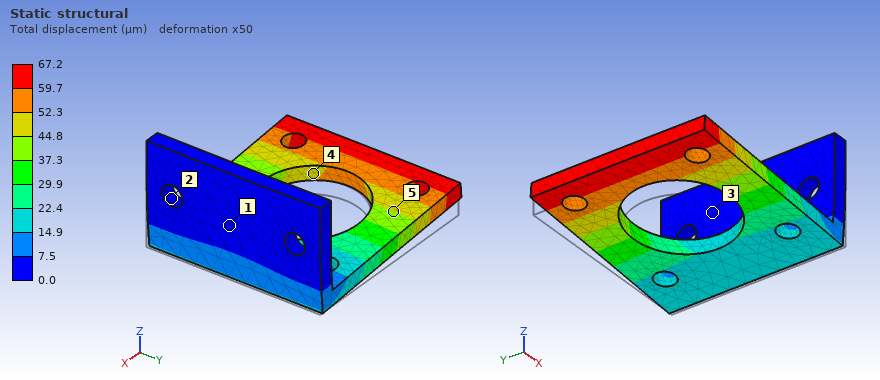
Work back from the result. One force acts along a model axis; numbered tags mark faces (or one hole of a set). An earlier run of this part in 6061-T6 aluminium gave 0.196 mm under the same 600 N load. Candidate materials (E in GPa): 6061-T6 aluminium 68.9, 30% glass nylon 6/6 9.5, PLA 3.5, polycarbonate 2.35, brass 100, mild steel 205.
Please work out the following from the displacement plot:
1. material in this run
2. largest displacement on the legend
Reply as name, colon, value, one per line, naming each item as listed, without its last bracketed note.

material in this run: mild steel
largest displacement on the legend: 67.2 µm
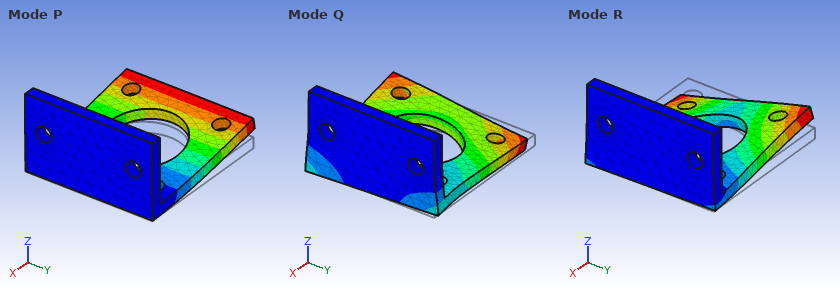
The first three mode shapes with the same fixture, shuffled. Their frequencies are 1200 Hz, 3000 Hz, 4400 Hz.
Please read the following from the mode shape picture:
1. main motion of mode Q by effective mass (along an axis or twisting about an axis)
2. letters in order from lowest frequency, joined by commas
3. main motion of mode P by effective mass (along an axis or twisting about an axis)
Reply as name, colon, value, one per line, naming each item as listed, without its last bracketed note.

main motion of mode Q by effective mass: along Y
letters in order from lowest frequency, joined by commas: P, R, Q
main motion of mode P by effective mass: along Z
